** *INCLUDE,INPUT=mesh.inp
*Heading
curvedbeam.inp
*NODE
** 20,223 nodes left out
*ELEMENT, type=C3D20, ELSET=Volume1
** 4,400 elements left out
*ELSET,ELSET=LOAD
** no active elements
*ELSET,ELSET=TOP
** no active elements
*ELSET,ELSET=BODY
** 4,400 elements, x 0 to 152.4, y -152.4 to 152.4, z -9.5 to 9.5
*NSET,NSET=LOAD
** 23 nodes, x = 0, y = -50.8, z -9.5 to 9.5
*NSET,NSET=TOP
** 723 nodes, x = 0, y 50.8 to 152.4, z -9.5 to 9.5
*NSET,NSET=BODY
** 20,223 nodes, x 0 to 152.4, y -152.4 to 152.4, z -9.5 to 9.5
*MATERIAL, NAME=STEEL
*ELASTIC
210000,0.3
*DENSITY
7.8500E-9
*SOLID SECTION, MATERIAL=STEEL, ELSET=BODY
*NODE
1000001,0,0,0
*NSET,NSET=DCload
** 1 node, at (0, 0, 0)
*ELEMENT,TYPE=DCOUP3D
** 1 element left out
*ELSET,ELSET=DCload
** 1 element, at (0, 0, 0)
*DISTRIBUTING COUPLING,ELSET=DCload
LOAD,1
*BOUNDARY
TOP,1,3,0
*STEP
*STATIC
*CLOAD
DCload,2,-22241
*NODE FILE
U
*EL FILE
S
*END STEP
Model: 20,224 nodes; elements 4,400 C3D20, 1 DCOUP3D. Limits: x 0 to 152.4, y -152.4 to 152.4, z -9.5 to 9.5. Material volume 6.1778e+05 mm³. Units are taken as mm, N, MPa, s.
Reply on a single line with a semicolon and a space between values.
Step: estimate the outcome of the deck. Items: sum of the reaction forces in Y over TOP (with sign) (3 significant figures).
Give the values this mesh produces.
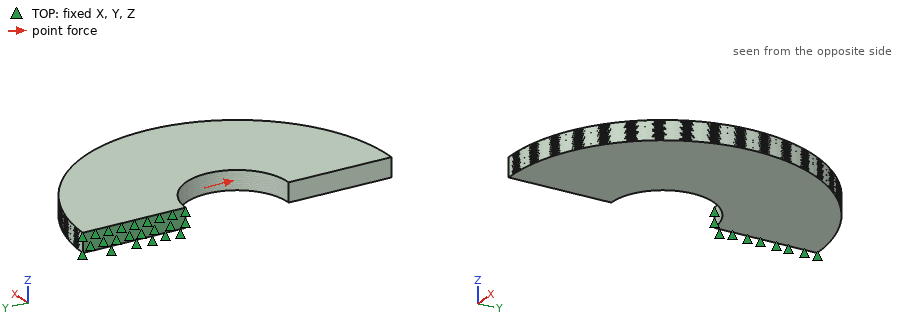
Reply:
22200 N
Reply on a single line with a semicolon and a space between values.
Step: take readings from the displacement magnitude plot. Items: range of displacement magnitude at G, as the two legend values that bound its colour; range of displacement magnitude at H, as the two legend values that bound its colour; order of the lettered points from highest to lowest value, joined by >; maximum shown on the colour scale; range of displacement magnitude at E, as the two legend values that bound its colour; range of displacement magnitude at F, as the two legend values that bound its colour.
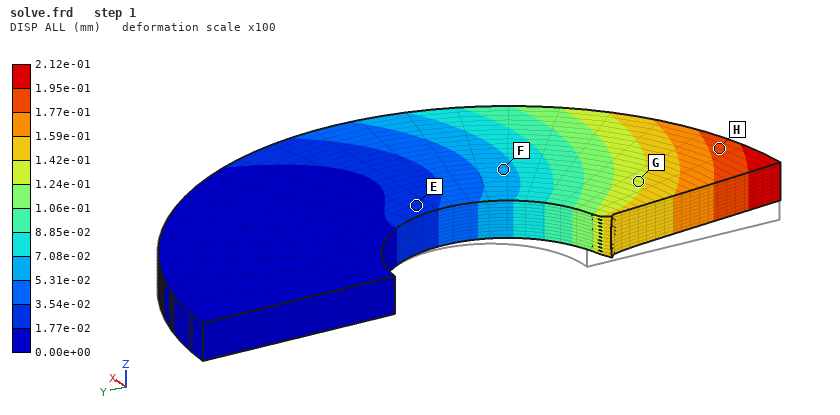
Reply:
1.24e-01 to 1.42e-01 mm; 1.77e-01 to 1.95e-01 mm; H > G > F > E; 2.12e-01 mm; 1.77e-02 to 3.54e-02 mm; 5.31e-02 to 7.08e-02 mm
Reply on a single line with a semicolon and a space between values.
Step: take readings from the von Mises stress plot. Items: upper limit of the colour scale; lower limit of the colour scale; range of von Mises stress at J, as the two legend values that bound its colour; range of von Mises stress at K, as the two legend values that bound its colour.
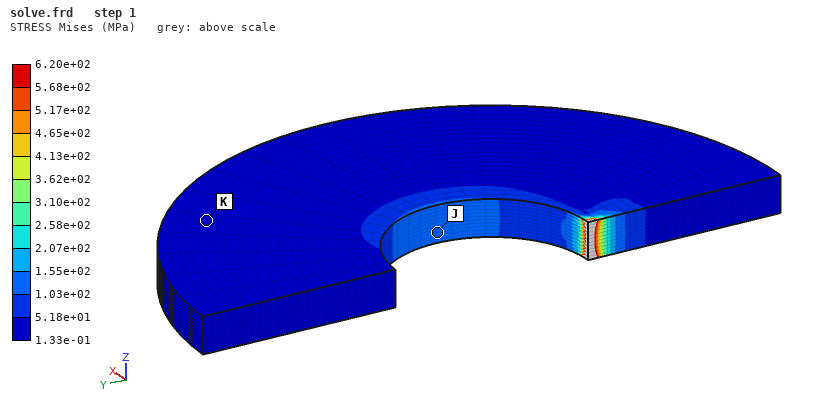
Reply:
6.20e+02 MPa; 1.33e-01 MPa; 1.03e+02 to 1.55e+02 MPa; 1.33e-01 to 5.18e+01 MPa
